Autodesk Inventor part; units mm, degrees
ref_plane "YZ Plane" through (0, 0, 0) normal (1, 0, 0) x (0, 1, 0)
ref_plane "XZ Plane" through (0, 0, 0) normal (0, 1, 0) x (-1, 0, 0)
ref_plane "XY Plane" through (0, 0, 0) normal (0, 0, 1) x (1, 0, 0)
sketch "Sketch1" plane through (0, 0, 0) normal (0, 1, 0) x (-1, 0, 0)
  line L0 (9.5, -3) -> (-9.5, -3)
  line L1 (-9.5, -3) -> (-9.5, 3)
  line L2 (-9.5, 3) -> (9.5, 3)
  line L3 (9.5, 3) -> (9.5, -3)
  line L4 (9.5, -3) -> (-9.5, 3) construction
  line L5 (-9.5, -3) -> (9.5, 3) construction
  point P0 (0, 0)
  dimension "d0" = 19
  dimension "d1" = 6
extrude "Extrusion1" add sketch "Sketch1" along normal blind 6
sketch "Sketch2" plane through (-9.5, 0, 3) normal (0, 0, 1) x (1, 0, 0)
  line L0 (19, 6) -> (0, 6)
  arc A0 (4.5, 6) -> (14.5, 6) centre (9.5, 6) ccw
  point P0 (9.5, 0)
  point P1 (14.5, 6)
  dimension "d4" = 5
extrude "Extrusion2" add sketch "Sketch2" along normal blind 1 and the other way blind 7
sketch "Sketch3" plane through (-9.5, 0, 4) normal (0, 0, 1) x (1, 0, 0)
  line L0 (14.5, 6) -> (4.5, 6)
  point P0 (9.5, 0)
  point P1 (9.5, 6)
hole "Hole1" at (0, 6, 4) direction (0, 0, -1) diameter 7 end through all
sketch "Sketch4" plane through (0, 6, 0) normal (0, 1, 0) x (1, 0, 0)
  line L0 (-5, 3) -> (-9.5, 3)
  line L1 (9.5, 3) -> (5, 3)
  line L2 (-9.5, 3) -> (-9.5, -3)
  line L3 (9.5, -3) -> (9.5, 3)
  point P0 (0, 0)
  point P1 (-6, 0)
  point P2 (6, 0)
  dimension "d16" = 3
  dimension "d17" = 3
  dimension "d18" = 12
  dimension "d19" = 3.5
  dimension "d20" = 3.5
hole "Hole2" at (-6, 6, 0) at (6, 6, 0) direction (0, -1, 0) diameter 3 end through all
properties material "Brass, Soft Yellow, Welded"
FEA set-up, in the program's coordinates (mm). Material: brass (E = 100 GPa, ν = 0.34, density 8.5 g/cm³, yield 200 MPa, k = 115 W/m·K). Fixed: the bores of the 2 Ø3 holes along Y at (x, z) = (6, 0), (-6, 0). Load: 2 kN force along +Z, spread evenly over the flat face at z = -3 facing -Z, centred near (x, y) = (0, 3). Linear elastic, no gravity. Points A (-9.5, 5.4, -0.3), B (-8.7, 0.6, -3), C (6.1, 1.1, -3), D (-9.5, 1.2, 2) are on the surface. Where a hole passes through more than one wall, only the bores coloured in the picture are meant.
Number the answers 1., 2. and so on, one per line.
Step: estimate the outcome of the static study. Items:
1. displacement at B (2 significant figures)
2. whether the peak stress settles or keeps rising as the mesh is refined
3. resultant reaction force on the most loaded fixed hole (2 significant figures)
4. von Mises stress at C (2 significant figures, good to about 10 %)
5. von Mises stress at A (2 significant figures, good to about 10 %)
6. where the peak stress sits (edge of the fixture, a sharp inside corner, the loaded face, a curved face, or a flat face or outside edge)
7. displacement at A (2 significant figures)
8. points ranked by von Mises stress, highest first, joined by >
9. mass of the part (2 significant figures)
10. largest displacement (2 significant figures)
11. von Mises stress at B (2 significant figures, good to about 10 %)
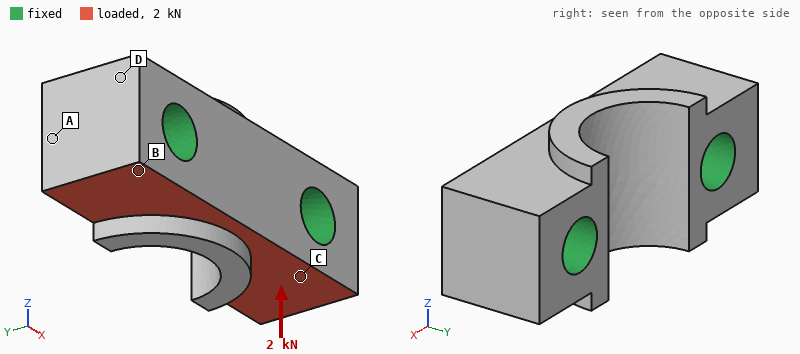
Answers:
1. 1.4 µm
2. keeps rising
3. 1.0 kN
4. 44 MPa
5. 18 MPa
6. edge of the fixture
7. 0.75 µm
8. C > B > A > D
9. 4.5 g
10. 1.8 µm
11. 27 MPa
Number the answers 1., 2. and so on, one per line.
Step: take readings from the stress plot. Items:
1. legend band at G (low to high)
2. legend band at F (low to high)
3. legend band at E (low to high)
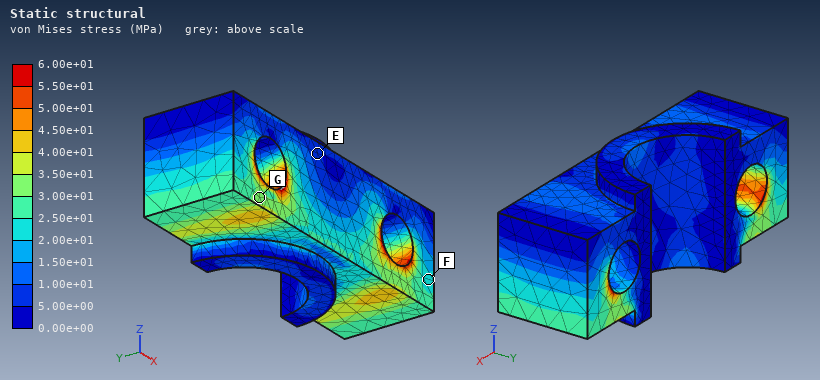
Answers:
1. 3.00e+01 to 3.50e+01 MPa
2. 2.00e+01 to 2.50e+01 MPa
3. 5.00e+00 to 1.00e+01 MPa
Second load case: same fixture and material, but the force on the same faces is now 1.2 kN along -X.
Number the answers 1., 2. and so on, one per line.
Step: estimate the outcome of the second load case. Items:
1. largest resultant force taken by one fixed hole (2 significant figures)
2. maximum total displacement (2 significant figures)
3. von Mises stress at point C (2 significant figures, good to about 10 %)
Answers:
1. 610 N
2. 2.2 µm
3. 30 MPa
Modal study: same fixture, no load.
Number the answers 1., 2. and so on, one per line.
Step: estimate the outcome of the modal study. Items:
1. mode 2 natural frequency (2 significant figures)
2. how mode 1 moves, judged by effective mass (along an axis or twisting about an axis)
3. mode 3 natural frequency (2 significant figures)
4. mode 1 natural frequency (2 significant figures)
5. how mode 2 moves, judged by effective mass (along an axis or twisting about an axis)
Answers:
1. 93 kHz
2. along Z
3. 110 kHz
4. 85 kHz
5. along Y
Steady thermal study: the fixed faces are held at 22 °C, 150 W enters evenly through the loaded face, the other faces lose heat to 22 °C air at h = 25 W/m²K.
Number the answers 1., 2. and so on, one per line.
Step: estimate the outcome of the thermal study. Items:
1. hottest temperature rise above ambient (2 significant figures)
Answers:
1. 43 K
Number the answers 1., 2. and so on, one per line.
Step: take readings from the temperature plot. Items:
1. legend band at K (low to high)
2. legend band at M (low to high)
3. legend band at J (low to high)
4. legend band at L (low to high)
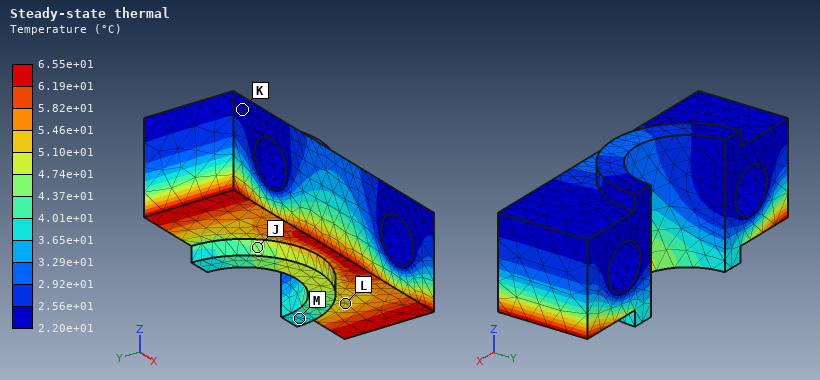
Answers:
1. 2.20e+01 to 2.56e+01 °C
2. 3.65e+01 to 4.01e+01 °C
3. 4.37e+01 to 4.74e+01 °C
4. 5.10e+01 to 5.46e+01 °C
